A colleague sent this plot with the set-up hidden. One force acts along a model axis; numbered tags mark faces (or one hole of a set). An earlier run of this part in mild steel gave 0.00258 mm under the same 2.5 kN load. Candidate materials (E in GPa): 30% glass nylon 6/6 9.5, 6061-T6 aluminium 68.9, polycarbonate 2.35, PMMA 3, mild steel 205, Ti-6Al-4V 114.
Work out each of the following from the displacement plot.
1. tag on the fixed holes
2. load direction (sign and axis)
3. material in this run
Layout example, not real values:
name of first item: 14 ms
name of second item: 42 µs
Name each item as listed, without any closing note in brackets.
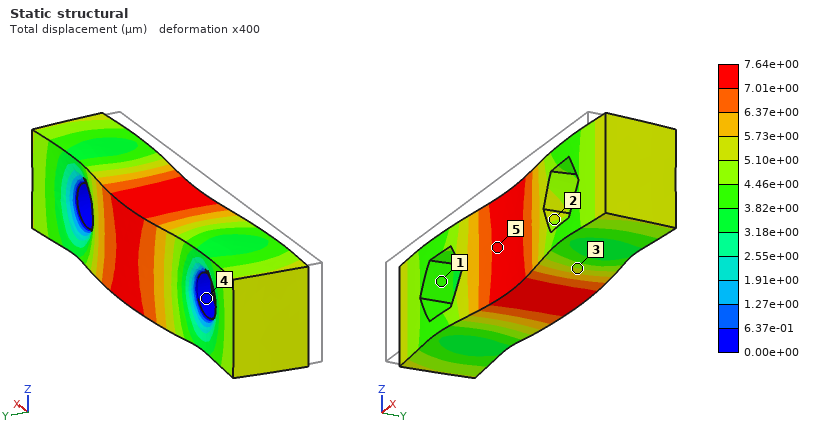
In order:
tag on the fixed holes: 4
load direction: +Y
material in this run: 6061-T6 aluminium
